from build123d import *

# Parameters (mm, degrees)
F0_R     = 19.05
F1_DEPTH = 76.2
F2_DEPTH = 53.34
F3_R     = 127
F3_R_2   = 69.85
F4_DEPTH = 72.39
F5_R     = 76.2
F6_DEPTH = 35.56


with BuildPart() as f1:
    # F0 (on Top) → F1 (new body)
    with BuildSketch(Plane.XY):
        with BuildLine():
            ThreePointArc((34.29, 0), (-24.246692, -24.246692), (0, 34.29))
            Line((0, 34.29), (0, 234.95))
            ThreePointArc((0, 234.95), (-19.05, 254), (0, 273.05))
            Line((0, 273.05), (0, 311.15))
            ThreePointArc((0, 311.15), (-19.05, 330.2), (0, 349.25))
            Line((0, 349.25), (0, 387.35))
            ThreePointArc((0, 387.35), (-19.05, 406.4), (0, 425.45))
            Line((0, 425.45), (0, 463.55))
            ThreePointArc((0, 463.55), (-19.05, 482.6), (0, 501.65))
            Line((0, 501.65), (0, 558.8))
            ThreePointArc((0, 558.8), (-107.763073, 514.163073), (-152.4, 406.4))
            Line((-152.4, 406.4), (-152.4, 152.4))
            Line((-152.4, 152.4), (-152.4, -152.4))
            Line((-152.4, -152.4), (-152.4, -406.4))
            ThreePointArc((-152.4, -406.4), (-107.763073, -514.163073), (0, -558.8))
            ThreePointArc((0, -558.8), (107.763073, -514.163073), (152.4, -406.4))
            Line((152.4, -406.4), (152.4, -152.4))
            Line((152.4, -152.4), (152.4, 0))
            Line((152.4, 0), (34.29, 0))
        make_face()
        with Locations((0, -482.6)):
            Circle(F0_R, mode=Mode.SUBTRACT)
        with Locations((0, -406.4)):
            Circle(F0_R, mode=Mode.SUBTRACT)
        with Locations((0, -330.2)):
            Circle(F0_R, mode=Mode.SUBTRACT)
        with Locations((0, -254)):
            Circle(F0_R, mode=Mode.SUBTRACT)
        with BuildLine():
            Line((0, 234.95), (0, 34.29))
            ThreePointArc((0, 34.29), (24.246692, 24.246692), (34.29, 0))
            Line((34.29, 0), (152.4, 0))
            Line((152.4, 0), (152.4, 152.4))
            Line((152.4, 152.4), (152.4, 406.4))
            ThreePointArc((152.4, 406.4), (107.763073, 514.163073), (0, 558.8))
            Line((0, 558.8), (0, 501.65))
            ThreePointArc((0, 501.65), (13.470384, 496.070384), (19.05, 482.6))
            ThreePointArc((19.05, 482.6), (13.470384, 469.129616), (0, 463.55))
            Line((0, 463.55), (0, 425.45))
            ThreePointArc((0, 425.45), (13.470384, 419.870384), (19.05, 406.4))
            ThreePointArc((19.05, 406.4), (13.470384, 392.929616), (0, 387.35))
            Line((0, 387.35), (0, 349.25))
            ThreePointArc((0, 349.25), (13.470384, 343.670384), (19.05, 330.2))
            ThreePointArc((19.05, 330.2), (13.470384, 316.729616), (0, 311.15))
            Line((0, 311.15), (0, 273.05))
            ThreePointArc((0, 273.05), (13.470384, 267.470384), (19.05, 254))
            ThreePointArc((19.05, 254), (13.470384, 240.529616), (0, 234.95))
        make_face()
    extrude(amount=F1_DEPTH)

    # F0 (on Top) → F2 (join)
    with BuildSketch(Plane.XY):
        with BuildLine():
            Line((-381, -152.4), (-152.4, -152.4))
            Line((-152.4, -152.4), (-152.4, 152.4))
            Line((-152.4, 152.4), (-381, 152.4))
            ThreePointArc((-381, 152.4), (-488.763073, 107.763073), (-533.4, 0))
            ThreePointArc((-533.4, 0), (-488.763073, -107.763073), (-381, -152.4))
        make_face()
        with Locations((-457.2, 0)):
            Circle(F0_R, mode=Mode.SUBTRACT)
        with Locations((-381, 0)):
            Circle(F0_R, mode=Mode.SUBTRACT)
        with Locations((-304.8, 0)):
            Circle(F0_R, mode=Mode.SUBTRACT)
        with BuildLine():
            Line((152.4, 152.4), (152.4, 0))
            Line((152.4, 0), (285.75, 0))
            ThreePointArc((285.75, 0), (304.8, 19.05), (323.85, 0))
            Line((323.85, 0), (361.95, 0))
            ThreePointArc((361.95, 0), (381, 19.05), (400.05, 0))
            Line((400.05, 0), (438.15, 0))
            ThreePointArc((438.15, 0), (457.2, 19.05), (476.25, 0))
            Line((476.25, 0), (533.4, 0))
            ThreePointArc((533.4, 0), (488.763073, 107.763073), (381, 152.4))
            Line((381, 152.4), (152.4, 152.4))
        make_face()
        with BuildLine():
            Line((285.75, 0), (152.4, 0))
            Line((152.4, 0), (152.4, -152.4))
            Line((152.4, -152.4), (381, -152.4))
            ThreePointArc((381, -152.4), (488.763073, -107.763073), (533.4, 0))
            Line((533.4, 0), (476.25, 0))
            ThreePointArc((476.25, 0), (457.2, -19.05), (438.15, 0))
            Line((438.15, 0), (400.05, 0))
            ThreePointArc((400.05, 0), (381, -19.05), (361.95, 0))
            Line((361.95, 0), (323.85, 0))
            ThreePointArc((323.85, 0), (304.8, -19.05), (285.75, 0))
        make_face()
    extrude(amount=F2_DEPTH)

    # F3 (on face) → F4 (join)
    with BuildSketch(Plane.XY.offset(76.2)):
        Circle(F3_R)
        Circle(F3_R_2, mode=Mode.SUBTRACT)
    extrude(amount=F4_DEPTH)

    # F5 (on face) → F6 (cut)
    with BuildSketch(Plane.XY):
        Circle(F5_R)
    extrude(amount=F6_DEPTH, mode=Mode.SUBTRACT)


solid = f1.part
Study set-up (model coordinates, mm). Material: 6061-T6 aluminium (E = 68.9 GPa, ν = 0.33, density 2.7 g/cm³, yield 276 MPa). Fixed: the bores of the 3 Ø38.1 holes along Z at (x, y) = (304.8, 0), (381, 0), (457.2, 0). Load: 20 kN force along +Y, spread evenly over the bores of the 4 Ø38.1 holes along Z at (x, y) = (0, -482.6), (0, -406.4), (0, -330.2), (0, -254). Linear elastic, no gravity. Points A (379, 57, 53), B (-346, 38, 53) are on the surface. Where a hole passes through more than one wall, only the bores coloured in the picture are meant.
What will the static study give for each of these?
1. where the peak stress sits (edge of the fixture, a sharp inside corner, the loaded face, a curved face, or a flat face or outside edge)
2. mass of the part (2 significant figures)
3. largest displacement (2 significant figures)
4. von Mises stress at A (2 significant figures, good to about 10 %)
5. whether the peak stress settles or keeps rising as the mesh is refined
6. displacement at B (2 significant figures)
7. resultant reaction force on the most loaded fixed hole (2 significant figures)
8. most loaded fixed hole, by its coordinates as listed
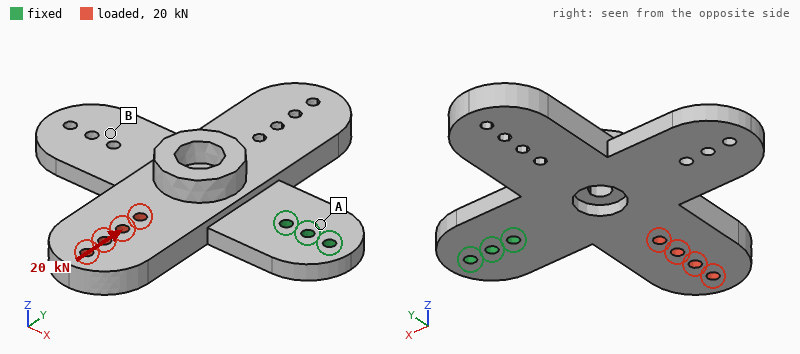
edge of the fixture
98 kg
0.22 mm
4.3 MPa
keeps rising
0.17 mm
51 kN
(304.8, 0)
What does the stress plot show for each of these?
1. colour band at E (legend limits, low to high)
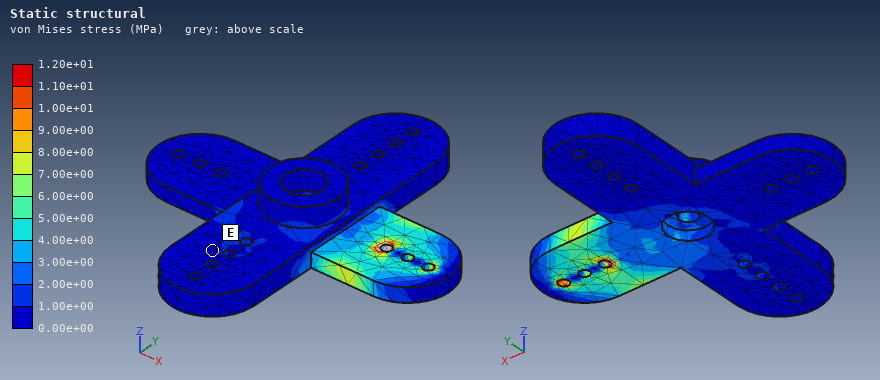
0.00e+00 to 1.00e+00 MPa
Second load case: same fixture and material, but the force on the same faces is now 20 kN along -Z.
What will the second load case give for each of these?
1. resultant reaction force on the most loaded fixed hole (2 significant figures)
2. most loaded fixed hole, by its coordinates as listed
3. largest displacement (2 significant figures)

45 kN
(304.8, 0)
3.3 mm
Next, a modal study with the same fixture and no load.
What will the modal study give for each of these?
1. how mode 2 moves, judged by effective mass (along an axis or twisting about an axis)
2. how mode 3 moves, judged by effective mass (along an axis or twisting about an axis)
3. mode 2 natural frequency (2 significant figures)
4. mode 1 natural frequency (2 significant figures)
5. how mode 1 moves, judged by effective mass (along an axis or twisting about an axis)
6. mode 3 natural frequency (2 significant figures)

twisting about X
along Y
91 Hz
63 Hz
along Z
170 Hz
